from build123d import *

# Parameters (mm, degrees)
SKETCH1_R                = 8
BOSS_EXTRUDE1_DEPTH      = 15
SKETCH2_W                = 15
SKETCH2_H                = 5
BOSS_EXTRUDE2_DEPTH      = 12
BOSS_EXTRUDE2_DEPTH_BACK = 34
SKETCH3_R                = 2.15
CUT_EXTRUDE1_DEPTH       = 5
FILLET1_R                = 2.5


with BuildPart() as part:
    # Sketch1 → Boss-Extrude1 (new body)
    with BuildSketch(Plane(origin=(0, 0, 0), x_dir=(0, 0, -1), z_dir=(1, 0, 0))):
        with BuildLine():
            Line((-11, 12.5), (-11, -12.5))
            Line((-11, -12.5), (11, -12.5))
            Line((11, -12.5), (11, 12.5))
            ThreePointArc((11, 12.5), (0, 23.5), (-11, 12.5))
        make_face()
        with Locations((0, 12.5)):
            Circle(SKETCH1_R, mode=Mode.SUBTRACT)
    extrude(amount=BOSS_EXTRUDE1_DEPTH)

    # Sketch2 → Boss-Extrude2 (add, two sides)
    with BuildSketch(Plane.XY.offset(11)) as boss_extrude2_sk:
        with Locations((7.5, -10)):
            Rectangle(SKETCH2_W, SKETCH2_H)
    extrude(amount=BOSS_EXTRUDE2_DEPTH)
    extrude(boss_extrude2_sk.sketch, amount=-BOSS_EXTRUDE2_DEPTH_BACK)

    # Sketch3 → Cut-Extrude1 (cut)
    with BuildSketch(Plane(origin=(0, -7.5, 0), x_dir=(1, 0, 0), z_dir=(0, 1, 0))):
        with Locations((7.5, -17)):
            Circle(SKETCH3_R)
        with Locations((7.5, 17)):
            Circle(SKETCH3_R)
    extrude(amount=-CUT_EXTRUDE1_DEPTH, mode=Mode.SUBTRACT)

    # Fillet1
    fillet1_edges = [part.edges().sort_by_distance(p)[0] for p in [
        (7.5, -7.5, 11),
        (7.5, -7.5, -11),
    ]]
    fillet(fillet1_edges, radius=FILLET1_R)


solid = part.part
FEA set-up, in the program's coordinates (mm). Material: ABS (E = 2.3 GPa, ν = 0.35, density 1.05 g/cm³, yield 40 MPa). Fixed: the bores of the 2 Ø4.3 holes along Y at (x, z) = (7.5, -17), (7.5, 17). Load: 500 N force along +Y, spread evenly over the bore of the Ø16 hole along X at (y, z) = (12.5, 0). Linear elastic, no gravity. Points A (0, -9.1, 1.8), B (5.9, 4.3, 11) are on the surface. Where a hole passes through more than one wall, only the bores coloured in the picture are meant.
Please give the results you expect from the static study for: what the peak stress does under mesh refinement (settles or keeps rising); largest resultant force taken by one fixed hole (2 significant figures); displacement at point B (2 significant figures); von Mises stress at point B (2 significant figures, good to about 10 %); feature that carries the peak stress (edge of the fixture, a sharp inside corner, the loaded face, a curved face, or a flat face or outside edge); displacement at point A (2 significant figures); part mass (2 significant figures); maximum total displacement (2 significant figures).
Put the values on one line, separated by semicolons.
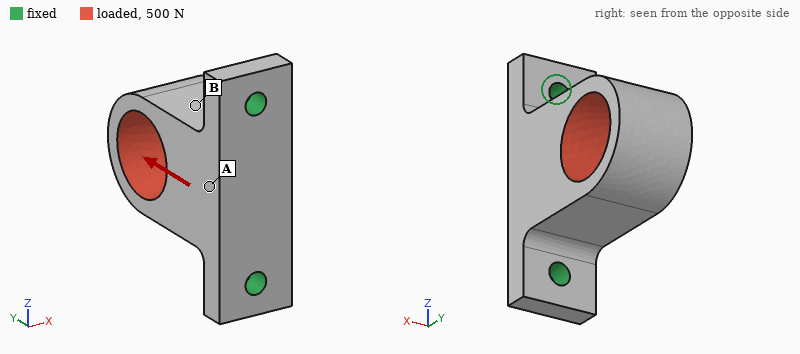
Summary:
keeps rising; 270 N; 0.073 mm; 4.5 MPa; edge of the fixture; 0.064 mm; 10 g; 0.14 mm
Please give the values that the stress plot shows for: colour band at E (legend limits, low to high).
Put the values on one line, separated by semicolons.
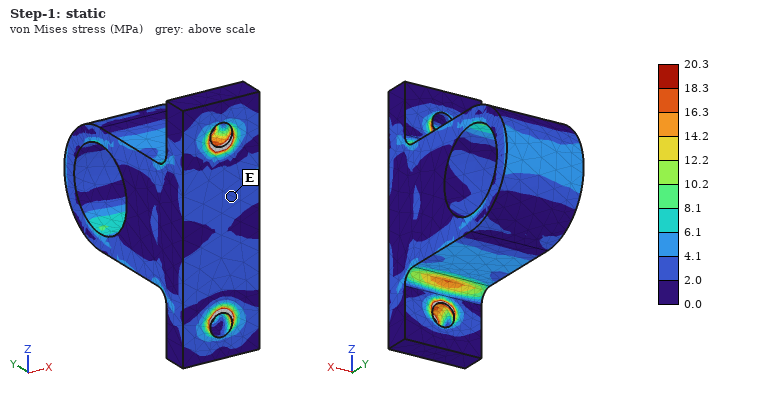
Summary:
2.0 to 4.1 MPa
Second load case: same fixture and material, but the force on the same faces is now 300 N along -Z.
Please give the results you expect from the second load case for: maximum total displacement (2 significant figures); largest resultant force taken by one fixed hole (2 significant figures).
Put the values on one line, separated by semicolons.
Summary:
0.37 mm; 280 N
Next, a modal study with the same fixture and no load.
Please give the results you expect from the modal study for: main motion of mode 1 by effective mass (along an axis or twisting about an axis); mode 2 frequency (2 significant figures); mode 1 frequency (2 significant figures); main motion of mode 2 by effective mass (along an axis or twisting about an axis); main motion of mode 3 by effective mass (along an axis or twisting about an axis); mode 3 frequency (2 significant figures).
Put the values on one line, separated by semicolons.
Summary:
along X; 2900 Hz; 1400 Hz; along Z; along Y; 4800 Hz
